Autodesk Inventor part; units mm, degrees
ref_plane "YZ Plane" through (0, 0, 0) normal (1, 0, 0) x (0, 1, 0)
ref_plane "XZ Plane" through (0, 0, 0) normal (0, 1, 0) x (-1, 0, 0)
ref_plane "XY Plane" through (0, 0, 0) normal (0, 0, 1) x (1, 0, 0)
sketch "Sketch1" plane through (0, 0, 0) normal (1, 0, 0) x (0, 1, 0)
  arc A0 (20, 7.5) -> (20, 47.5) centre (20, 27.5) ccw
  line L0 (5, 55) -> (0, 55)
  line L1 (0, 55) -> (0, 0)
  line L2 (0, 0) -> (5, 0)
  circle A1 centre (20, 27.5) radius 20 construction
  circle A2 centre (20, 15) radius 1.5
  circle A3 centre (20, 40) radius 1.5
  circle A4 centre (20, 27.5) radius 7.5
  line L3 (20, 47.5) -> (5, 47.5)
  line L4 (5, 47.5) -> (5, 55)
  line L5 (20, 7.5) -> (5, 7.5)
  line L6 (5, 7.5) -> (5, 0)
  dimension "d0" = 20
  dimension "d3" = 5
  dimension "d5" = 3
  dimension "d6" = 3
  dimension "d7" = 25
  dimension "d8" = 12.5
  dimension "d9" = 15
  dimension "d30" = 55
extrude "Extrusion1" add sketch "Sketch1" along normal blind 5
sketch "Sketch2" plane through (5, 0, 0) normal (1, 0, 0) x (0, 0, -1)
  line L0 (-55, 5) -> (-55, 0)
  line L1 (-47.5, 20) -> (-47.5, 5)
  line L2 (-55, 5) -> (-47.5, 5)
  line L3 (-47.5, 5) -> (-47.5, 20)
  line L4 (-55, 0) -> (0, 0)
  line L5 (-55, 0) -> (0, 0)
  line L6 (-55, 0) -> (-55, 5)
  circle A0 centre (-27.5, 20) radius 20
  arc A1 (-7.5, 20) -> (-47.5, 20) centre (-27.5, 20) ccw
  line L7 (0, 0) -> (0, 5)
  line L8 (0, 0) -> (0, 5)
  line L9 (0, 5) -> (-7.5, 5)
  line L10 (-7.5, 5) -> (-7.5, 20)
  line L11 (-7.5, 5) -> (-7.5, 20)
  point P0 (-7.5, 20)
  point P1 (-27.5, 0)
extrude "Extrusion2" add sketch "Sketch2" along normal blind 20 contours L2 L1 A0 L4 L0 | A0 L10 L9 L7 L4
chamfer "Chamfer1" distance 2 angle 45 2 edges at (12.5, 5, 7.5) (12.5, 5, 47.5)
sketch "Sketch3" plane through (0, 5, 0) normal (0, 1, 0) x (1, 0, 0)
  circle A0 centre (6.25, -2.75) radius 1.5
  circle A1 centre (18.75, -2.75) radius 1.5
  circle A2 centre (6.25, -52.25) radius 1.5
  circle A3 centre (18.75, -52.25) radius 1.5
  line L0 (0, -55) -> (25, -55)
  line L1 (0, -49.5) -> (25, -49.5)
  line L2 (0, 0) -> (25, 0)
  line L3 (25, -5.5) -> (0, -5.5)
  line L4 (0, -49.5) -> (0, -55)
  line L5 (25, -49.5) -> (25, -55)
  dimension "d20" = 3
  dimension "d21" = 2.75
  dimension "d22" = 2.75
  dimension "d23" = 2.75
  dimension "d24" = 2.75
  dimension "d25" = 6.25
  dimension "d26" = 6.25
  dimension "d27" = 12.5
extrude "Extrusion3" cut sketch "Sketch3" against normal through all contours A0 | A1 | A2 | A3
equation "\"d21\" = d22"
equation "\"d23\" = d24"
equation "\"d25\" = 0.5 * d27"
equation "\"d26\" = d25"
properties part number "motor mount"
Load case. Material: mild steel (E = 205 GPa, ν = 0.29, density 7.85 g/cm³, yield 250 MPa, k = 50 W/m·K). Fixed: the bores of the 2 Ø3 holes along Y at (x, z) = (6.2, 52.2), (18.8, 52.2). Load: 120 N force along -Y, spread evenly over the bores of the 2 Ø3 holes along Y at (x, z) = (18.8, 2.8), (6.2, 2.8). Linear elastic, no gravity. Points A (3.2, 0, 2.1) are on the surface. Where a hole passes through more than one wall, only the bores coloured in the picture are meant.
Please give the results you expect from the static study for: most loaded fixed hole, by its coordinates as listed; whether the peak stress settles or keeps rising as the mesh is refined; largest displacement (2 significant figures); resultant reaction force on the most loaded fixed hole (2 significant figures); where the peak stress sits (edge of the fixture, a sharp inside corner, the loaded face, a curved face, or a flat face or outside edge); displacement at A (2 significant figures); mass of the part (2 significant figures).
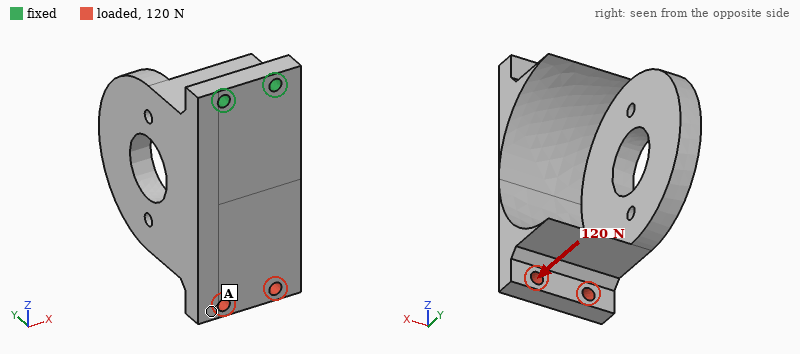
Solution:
(18.8, 52.2)
keeps rising
68 µm
76 N
edge of the fixture
53 µm
90 g
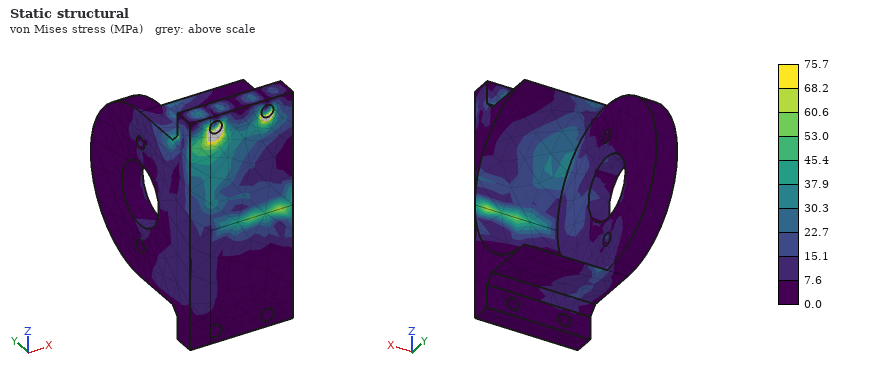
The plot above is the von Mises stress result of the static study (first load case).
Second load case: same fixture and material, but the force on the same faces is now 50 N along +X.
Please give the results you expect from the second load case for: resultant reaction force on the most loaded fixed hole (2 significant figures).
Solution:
170 N
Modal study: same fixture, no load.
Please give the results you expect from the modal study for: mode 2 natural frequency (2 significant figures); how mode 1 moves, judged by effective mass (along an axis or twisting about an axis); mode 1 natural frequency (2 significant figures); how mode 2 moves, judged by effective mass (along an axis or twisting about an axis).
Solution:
1700 Hz
along Y
1300 Hz
along X
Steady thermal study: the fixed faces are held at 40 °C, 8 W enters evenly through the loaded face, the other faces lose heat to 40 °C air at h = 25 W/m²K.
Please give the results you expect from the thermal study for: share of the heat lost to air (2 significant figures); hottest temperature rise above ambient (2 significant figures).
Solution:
51 %
57 K
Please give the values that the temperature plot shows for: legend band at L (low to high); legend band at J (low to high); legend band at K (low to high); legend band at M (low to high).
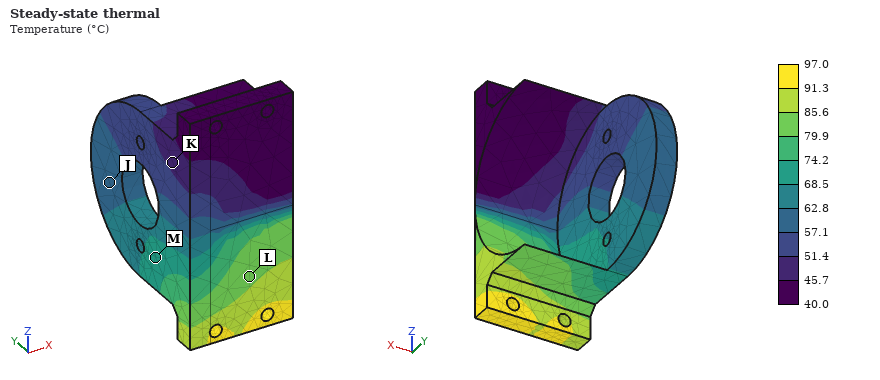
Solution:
79.9 to 85.6 °C
57.1 to 62.8 °C
45.7 to 51.4 °C
68.5 to 74.2 °C
